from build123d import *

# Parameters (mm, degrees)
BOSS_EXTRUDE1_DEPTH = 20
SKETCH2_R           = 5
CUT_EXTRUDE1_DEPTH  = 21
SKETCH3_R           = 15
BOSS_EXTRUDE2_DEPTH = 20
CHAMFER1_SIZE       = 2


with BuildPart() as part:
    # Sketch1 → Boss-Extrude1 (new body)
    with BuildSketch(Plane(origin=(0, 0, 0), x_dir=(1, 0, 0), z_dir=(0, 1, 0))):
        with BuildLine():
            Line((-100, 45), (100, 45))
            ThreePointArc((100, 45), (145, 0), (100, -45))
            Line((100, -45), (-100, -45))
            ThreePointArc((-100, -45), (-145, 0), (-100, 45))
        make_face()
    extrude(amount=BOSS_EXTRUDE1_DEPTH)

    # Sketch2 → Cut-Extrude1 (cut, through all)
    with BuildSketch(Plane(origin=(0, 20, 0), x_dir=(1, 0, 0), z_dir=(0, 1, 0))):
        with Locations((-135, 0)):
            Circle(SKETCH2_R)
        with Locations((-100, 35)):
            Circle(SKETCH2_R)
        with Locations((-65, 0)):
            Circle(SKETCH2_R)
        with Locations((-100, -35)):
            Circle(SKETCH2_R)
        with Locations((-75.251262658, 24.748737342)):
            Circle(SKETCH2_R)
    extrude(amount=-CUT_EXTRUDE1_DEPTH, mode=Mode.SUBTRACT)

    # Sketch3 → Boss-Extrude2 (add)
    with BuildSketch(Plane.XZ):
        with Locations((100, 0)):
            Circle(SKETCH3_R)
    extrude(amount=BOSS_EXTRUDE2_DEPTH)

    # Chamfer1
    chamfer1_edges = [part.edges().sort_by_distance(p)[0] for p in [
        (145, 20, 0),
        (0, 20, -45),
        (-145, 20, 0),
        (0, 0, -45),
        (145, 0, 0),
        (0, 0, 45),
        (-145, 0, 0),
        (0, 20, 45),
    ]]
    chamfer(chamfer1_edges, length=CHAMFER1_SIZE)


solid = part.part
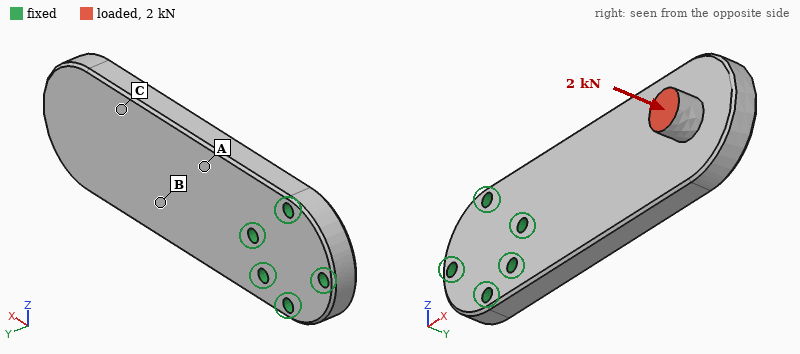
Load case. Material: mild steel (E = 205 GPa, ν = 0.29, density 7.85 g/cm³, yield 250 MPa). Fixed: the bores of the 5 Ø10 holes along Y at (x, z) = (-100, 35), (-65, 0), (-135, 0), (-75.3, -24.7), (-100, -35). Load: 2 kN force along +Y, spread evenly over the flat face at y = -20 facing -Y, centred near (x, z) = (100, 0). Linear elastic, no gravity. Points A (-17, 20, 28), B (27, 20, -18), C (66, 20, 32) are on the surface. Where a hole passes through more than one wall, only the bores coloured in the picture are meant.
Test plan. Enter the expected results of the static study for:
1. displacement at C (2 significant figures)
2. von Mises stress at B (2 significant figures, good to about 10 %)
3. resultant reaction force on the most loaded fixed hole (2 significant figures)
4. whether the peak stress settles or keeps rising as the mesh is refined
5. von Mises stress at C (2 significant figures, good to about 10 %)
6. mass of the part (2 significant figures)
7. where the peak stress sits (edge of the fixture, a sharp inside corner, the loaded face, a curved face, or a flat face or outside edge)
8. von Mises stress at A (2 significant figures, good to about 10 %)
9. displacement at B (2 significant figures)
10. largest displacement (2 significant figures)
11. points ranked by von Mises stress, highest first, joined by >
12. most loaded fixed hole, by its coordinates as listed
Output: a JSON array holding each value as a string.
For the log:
["0.19 mm", "24 MPa", "5.8 kN", "keeps rising", "12 MPa", "3.9 kg", "edge of the fixture", "38 MPa", "0.10 mm", "0.37 mm", "A > B > C", "(-65, 0)"]
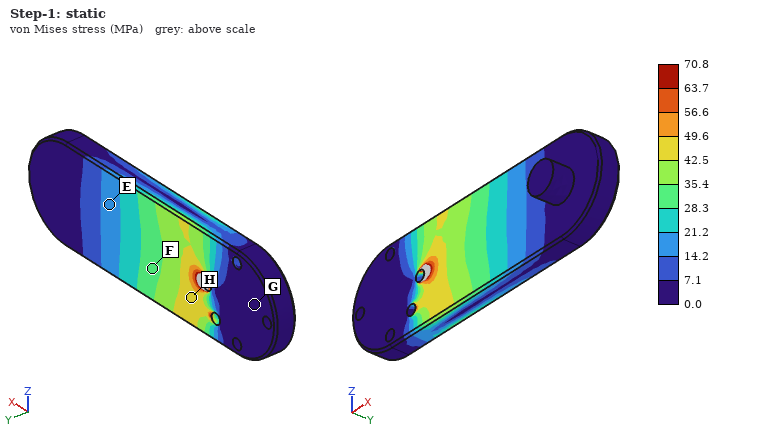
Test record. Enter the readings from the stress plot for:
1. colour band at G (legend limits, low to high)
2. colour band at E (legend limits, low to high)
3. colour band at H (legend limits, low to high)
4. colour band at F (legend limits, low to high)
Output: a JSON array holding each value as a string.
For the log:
["0.0 to 7.1 MPa", "14.2 to 21.2 MPa", "42.5 to 49.6 MPa", "28.3 to 35.4 MPa"]
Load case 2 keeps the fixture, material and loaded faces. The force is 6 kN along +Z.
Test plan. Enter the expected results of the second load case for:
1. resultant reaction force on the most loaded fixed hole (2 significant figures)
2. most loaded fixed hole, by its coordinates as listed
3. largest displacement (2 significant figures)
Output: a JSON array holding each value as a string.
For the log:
["13 kN", "(-75.3, -24.7)", "0.12 mm"]
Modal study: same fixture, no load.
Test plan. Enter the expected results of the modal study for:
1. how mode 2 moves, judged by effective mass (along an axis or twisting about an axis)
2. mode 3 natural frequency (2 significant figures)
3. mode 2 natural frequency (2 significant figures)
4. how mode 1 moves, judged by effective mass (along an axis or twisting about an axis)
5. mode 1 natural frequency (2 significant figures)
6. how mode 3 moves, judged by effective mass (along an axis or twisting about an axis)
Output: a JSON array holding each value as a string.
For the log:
["along Z", "1700 Hz", "1300 Hz", "along Y", "380 Hz", "twisting about X"]
